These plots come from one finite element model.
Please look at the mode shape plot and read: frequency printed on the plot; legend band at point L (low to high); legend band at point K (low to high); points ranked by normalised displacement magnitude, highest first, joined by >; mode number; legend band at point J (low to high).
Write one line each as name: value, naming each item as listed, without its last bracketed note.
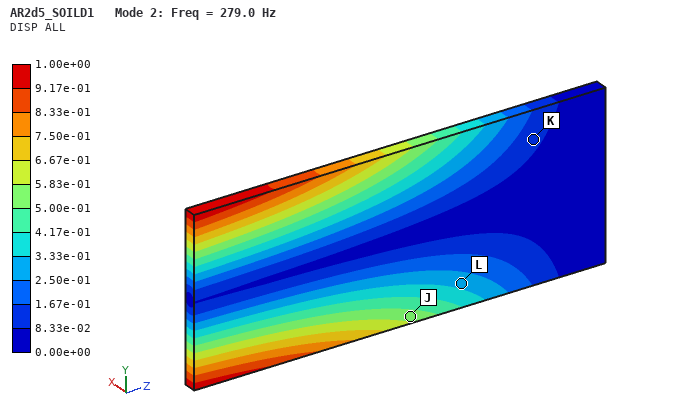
frequency printed on the plot: 279.0 Hz
legend band at point L: 2.50e-01 to 3.33e-01
legend band at point K: 8.33e-02 to 1.67e-01
points ranked by normalised displacement magnitude, highest first, joined by >: J > L > K
mode number: 2
legend band at point J: 5.00e-01 to 5.83e-01
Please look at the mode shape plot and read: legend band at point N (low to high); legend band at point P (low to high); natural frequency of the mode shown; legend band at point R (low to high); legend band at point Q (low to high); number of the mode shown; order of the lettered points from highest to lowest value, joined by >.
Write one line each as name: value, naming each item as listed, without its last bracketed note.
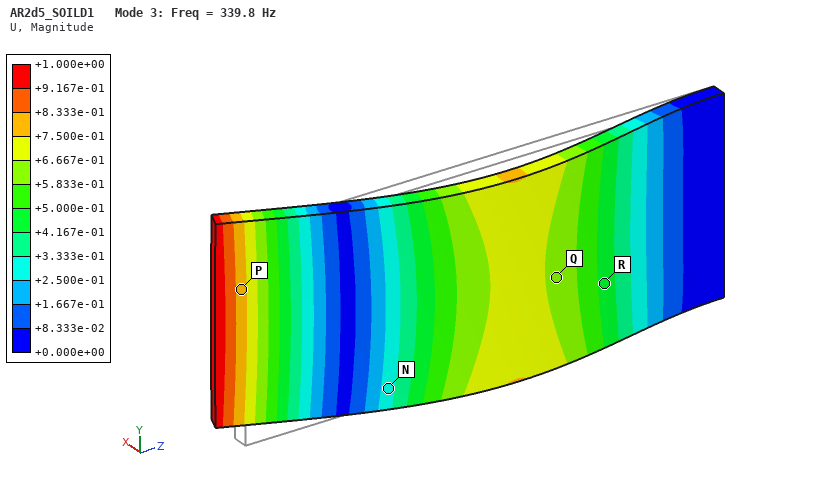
legend band at point N: +2.500e-01 to +3.333e-01
legend band at point P: +7.500e-01 to +8.333e-01
natural frequency of the mode shown: 339.8 Hz
legend band at point R: +4.167e-01 to +5.000e-01
legend band at point Q: +5.833e-01 to +6.667e-01
number of the mode shown: 3
order of the lettered points from highest to lowest value, joined by >: P > Q > R > N
